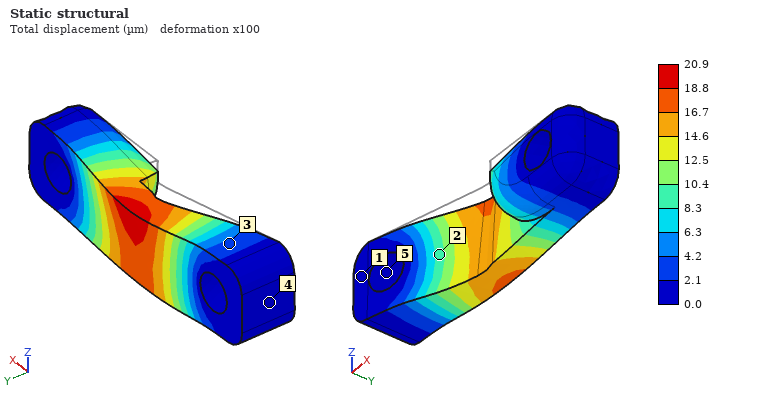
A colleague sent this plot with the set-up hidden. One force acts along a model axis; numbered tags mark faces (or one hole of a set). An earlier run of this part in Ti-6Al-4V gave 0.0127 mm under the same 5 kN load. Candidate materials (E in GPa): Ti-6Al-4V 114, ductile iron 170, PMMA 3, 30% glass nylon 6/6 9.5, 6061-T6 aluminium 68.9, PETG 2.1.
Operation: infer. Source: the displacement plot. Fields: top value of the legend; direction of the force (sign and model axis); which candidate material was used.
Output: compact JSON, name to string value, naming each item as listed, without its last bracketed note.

{"top value of the legend": "20.9 µm", "direction of the force": "-Z", "which candidate material was used": "6061-T6 aluminium"}
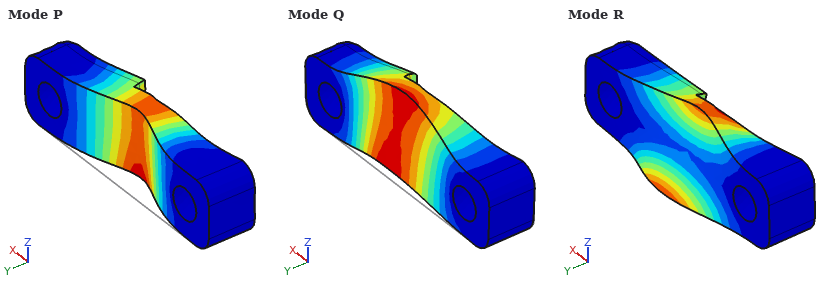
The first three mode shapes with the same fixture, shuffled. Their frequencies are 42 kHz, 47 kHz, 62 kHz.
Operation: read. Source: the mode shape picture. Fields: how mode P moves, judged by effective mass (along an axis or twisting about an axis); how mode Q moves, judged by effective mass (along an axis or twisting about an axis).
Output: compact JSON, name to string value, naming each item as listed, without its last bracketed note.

{"how mode P moves, judged by effective mass": "along Y", "how mode Q moves, judged by effective mass": "along Z"}
